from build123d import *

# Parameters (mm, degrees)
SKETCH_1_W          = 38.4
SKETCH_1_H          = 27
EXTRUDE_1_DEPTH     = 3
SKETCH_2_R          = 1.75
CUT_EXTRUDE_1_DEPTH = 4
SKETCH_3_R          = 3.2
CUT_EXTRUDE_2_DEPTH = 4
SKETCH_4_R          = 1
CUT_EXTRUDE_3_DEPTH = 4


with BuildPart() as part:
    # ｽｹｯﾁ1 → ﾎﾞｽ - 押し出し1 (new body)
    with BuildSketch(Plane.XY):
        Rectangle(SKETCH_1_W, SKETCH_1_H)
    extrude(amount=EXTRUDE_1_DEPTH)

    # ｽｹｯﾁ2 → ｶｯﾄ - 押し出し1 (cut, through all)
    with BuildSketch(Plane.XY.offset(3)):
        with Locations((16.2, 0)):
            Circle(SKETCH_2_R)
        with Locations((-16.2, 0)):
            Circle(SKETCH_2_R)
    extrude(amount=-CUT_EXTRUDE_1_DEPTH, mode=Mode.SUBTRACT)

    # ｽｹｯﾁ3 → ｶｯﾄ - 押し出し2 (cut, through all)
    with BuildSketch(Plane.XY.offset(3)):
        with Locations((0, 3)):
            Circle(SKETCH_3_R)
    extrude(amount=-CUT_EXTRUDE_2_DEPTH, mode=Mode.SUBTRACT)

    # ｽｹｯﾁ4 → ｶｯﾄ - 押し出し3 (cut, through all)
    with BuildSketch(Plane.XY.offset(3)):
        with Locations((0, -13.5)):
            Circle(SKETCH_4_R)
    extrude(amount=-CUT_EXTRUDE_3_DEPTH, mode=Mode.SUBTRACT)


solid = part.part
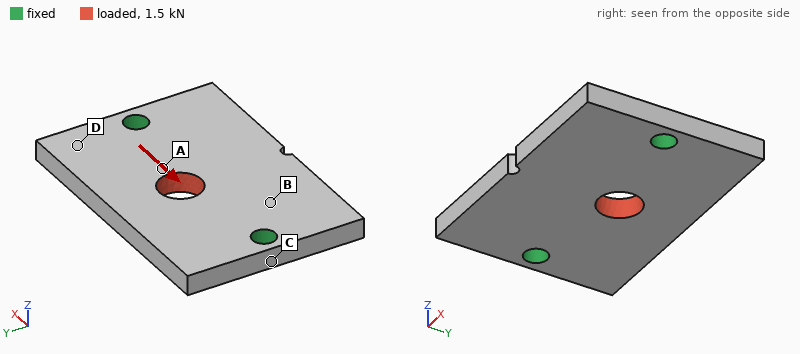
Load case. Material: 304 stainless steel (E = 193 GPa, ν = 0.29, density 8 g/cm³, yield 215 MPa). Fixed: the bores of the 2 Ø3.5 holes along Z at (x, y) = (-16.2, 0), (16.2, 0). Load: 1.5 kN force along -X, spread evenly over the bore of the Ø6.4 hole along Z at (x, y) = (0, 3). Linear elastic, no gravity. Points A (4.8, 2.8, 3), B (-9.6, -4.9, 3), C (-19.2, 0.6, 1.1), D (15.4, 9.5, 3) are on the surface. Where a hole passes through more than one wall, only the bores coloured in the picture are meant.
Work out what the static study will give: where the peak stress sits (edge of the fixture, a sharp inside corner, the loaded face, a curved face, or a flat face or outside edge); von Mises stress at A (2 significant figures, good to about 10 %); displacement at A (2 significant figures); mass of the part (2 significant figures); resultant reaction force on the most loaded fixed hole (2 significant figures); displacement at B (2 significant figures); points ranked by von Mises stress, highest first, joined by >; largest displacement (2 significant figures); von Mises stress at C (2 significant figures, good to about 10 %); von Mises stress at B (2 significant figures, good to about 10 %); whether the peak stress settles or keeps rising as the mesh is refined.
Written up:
edge of the fixture
28 MPa
1.6 µm
24 g
760 N
0.72 µm
A > C > B > D
2.3 µm
23 MPa
9.1 MPa
keeps rising
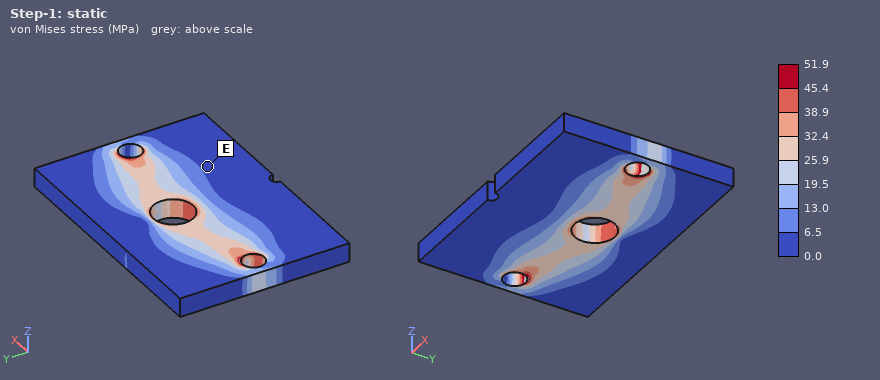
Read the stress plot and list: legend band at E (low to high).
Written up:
0.0 to 6.5 MPa
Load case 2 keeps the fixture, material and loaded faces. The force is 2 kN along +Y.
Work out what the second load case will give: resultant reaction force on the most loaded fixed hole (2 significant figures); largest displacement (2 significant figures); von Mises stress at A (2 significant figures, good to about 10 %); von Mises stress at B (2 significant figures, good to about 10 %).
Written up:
1.0 kN
5.0 µm
36 MPa
27 MPa
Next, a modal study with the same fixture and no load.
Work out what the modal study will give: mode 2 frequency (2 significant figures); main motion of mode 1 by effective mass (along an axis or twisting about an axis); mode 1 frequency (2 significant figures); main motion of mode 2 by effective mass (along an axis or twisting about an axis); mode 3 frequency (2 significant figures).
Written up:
10000 Hz
twisting about X
8300 Hz
along Z
16 kHz
